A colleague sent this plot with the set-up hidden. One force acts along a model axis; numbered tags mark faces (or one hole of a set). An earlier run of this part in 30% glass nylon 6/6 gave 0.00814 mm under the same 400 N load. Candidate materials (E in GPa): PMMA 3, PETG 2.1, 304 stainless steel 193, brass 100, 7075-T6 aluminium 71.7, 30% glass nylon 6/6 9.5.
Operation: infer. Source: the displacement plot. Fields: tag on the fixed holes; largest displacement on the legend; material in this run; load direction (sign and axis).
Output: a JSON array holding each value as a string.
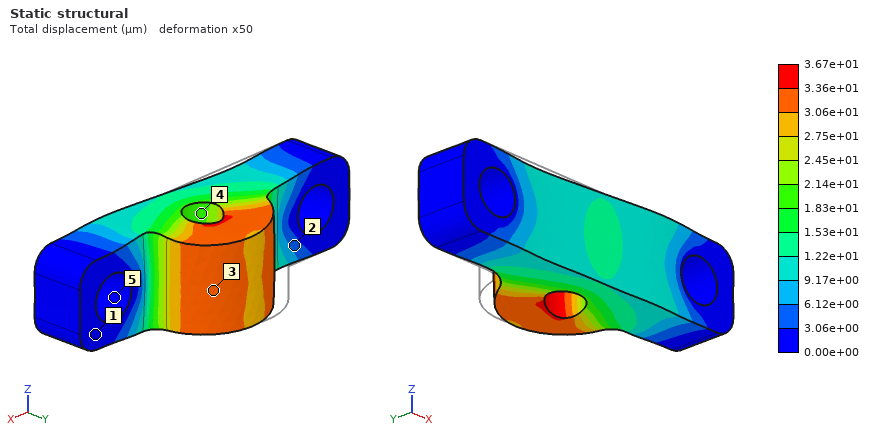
["5", "3.67e+01 µm", "PETG", "+X"]
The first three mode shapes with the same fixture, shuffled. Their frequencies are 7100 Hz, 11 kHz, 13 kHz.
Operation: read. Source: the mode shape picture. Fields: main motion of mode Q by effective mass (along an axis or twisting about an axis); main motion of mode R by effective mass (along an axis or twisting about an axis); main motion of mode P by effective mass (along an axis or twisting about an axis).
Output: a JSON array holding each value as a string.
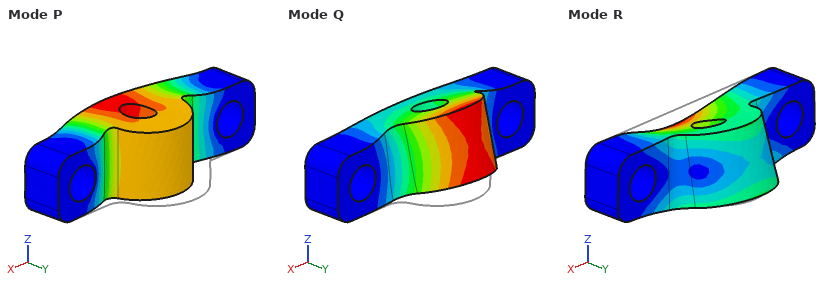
["along Z", "along Z", "along Y"]
